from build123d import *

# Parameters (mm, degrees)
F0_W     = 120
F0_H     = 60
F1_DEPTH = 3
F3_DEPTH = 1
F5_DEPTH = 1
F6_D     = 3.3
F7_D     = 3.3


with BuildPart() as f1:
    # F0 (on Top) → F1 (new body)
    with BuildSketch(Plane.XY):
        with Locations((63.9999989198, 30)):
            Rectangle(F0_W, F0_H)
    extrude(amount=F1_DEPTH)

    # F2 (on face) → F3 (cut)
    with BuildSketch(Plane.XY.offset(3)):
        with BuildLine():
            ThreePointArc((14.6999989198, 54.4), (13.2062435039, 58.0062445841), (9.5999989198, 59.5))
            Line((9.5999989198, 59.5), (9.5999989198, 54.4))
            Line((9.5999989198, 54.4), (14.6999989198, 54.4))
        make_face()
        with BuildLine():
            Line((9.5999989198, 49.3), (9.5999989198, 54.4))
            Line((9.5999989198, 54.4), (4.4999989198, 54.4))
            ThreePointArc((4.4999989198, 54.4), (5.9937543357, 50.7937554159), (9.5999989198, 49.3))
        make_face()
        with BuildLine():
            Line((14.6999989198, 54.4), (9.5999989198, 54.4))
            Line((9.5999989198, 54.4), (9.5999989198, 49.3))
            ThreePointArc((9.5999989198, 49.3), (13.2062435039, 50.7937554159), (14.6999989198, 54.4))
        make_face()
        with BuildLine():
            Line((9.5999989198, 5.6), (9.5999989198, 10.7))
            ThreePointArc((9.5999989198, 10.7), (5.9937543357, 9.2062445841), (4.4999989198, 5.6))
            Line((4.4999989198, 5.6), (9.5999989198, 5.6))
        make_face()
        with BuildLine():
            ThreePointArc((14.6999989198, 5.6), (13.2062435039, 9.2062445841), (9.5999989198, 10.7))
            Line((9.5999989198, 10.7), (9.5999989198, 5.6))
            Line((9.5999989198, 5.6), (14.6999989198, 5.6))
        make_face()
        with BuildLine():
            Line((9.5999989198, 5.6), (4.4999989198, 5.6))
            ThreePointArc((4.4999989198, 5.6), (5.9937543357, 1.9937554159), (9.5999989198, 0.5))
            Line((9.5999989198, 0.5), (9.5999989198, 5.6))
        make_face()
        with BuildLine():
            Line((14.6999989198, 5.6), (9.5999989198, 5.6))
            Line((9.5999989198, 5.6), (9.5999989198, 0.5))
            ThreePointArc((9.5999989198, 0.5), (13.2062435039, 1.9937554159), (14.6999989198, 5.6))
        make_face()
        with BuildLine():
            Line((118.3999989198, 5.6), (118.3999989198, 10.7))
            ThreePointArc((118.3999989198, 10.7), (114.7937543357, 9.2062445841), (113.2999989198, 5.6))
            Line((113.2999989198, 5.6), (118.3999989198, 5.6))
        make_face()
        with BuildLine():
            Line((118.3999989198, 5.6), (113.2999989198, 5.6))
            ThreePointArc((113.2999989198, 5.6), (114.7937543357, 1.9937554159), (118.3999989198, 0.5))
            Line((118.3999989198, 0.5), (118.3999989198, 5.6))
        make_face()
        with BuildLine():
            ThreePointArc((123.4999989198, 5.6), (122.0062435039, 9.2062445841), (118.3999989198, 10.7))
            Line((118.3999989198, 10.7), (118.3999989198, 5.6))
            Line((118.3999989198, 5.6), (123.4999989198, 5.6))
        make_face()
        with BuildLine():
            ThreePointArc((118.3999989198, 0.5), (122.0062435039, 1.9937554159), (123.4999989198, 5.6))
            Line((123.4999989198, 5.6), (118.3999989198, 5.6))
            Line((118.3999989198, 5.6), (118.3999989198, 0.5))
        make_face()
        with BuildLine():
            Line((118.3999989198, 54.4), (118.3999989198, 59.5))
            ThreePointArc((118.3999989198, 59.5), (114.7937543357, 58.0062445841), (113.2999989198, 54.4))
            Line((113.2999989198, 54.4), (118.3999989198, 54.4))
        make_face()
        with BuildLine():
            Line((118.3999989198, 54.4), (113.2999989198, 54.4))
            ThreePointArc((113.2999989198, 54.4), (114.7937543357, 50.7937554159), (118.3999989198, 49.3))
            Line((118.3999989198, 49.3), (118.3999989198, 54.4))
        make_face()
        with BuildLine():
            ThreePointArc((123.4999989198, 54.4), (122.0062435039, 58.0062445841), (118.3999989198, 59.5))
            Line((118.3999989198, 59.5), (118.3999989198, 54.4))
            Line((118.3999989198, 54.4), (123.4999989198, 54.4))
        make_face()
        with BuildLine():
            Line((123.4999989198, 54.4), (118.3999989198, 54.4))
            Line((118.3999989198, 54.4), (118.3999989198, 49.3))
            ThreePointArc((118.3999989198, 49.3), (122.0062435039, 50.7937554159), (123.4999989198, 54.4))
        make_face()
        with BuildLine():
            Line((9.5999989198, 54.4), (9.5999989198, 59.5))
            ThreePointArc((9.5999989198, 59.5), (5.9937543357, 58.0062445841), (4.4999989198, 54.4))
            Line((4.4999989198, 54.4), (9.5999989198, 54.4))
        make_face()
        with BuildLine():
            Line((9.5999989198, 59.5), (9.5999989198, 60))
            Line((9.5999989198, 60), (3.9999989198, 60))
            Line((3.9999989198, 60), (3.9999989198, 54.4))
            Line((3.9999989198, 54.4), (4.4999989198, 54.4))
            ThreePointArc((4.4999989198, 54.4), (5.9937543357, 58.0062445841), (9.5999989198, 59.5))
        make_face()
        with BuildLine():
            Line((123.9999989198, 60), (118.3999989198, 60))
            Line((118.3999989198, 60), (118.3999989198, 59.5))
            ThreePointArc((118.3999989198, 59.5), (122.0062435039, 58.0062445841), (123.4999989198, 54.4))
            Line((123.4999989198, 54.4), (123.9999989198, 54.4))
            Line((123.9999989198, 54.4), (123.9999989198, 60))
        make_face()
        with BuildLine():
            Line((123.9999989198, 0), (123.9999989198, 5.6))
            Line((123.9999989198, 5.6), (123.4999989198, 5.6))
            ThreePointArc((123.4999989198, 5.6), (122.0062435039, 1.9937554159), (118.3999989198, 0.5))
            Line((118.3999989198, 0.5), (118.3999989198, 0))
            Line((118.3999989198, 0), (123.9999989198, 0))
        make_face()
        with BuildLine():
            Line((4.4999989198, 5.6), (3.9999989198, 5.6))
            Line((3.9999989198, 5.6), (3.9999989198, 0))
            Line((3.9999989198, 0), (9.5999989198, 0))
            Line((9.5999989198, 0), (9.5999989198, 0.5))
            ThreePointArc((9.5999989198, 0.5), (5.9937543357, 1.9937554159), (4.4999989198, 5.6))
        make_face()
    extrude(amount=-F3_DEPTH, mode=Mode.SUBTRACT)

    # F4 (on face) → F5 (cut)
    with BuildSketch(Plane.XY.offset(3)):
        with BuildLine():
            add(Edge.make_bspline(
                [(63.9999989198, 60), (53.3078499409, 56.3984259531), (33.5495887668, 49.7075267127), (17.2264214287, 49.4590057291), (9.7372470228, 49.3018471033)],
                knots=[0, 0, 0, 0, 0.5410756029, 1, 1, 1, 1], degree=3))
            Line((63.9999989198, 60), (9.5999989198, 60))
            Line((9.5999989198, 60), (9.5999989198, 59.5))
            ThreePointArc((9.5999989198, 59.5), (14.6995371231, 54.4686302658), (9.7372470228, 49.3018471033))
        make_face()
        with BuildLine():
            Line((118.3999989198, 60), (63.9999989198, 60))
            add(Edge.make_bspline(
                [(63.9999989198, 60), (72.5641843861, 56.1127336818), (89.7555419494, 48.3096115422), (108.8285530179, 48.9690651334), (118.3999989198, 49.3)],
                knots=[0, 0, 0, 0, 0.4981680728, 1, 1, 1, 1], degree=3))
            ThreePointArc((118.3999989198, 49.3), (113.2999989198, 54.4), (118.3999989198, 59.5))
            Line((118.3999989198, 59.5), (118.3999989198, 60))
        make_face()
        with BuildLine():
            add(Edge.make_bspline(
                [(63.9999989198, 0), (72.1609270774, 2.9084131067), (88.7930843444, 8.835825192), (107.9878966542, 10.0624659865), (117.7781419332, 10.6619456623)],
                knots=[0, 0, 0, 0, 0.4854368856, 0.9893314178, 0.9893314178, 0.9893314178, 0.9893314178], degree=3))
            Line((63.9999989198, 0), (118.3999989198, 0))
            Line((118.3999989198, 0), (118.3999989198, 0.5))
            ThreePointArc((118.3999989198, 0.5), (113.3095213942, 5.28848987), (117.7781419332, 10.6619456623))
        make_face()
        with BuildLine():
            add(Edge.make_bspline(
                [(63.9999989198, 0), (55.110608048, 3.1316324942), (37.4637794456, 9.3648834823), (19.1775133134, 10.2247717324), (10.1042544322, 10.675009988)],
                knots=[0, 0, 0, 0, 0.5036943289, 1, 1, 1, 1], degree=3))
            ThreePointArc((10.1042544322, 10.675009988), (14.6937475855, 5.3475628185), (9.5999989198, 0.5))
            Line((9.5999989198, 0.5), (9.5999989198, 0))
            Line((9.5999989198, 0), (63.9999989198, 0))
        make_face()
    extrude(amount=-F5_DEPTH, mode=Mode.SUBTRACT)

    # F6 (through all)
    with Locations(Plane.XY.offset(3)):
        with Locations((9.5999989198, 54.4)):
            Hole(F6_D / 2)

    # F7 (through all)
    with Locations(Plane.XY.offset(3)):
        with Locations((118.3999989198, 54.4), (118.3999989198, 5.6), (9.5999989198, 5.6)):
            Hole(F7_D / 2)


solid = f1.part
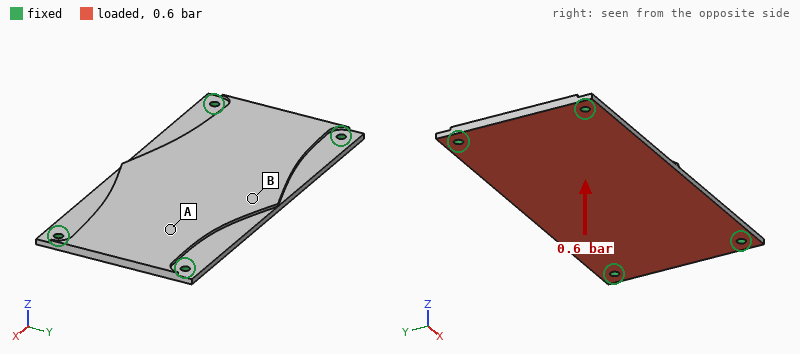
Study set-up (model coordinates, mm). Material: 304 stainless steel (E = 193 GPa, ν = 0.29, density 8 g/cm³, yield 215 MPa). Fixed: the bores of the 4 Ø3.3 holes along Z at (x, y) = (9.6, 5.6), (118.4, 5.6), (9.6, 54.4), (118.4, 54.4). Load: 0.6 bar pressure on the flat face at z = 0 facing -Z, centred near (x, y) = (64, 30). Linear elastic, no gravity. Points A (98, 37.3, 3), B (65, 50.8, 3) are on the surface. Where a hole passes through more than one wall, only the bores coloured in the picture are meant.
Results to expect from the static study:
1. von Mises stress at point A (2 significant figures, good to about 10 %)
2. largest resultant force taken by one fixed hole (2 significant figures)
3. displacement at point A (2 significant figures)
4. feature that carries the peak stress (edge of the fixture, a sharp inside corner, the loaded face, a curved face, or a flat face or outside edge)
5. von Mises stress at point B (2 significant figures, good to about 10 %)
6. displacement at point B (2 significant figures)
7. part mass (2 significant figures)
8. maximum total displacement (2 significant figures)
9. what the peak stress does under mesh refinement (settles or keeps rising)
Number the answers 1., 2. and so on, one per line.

1. 10 MPa
2. 230 N
3. 0.050 mm
4. edge of the fixture
5. 30 MPa
6. 0.10 mm
7. 160 g
8. 0.10 mm
9. keeps rising
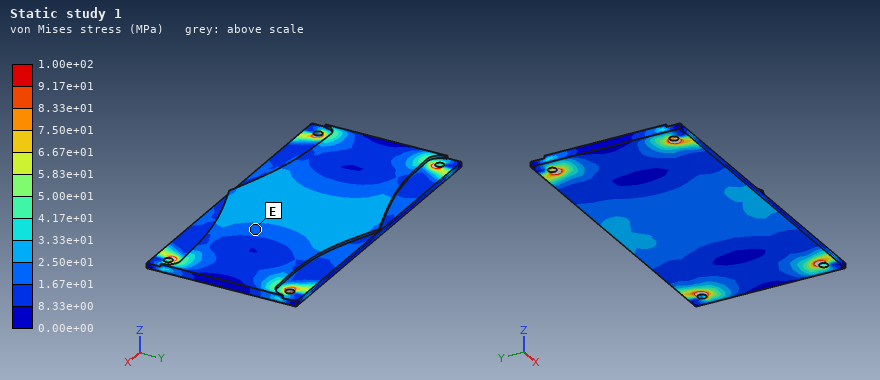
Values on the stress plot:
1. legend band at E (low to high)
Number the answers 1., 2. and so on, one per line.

1. 1.67e+01 to 2.50e+01 MPa
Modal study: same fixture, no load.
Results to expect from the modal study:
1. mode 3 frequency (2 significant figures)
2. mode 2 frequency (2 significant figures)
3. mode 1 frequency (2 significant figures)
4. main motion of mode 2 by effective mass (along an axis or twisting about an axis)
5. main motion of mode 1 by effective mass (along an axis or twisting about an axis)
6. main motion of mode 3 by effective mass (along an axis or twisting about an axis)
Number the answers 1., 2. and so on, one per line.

1. 2700 Hz
2. 1700 Hz
3. 930 Hz
4. twisting about X
5. along Z
6. twisting about Y
